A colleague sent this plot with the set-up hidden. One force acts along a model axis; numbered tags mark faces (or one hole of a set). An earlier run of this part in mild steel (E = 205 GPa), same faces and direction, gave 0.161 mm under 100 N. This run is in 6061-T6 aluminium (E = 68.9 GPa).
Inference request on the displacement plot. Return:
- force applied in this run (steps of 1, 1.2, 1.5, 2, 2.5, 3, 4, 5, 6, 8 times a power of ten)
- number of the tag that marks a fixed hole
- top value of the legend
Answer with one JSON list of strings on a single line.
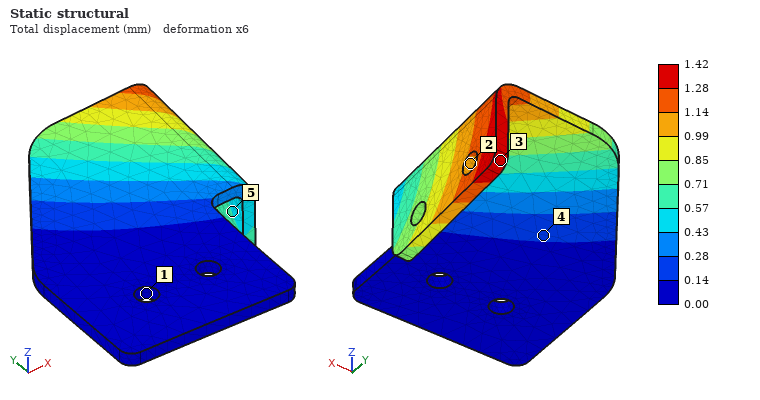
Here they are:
["300 N", "1", "1.42 mm"]
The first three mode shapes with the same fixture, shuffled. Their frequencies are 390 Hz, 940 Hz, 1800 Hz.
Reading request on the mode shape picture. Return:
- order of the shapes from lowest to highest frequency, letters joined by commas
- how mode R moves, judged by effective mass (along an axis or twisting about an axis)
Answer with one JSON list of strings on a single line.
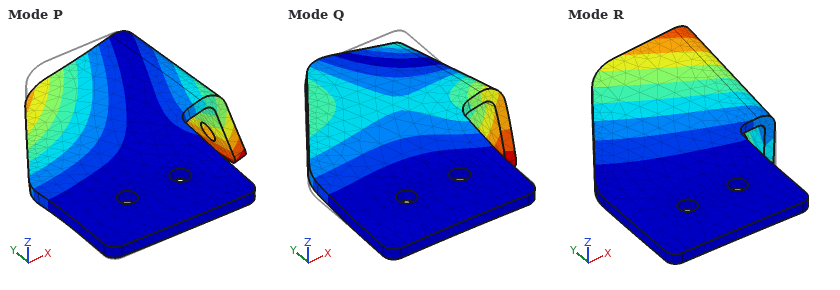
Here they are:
["R, P, Q", "along Z"]
